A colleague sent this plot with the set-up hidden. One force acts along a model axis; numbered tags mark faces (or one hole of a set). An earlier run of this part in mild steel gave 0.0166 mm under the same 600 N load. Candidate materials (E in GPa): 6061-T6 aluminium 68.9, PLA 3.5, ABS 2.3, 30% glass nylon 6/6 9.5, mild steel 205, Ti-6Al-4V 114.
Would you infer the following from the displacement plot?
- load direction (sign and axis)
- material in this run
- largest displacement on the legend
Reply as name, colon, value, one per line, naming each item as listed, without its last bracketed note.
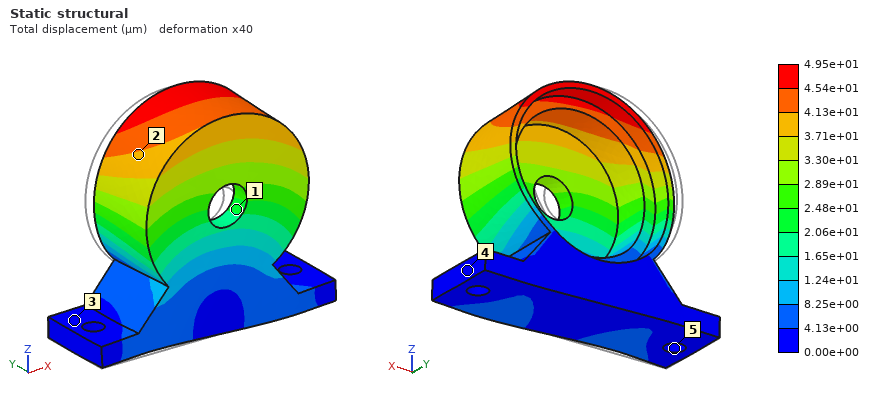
load direction: +X
material in this run: 6061-T6 aluminium
largest displacement on the legend: 4.95e+01 µm
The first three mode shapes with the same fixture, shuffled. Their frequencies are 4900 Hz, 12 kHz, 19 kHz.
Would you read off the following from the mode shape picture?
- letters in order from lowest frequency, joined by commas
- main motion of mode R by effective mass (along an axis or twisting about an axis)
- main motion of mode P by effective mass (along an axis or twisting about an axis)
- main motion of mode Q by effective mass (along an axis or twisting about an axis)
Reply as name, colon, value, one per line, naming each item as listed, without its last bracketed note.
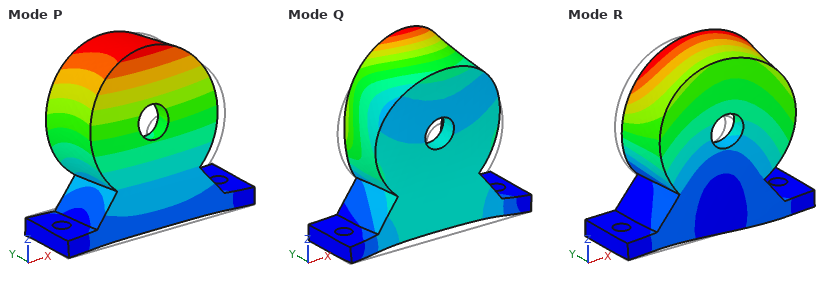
letters in order from lowest frequency, joined by commas: P, R, Q
main motion of mode R by effective mass: along X
main motion of mode P by effective mass: along Y
main motion of mode Q by effective mass: along Z
